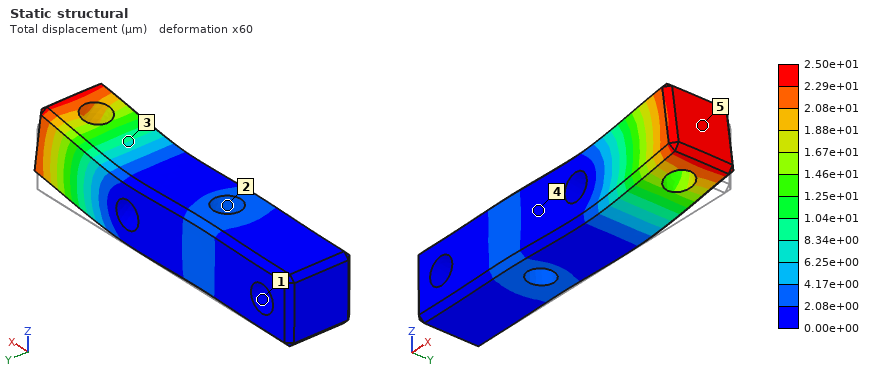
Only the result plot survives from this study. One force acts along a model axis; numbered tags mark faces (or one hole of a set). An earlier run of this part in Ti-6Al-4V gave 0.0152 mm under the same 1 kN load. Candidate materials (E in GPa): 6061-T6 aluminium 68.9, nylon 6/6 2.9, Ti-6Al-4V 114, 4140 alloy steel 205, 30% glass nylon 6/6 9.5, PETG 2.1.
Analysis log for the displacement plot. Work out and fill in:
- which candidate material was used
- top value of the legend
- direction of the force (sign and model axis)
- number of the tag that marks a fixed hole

6061-T6 aluminium
2.50e+01 µm
+Z
1
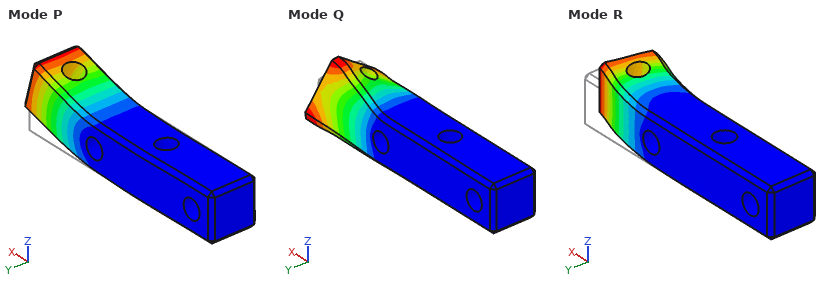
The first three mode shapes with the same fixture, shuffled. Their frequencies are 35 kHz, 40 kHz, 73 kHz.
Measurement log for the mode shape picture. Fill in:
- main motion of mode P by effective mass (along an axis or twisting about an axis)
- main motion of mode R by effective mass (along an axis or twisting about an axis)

along Z
along Y
